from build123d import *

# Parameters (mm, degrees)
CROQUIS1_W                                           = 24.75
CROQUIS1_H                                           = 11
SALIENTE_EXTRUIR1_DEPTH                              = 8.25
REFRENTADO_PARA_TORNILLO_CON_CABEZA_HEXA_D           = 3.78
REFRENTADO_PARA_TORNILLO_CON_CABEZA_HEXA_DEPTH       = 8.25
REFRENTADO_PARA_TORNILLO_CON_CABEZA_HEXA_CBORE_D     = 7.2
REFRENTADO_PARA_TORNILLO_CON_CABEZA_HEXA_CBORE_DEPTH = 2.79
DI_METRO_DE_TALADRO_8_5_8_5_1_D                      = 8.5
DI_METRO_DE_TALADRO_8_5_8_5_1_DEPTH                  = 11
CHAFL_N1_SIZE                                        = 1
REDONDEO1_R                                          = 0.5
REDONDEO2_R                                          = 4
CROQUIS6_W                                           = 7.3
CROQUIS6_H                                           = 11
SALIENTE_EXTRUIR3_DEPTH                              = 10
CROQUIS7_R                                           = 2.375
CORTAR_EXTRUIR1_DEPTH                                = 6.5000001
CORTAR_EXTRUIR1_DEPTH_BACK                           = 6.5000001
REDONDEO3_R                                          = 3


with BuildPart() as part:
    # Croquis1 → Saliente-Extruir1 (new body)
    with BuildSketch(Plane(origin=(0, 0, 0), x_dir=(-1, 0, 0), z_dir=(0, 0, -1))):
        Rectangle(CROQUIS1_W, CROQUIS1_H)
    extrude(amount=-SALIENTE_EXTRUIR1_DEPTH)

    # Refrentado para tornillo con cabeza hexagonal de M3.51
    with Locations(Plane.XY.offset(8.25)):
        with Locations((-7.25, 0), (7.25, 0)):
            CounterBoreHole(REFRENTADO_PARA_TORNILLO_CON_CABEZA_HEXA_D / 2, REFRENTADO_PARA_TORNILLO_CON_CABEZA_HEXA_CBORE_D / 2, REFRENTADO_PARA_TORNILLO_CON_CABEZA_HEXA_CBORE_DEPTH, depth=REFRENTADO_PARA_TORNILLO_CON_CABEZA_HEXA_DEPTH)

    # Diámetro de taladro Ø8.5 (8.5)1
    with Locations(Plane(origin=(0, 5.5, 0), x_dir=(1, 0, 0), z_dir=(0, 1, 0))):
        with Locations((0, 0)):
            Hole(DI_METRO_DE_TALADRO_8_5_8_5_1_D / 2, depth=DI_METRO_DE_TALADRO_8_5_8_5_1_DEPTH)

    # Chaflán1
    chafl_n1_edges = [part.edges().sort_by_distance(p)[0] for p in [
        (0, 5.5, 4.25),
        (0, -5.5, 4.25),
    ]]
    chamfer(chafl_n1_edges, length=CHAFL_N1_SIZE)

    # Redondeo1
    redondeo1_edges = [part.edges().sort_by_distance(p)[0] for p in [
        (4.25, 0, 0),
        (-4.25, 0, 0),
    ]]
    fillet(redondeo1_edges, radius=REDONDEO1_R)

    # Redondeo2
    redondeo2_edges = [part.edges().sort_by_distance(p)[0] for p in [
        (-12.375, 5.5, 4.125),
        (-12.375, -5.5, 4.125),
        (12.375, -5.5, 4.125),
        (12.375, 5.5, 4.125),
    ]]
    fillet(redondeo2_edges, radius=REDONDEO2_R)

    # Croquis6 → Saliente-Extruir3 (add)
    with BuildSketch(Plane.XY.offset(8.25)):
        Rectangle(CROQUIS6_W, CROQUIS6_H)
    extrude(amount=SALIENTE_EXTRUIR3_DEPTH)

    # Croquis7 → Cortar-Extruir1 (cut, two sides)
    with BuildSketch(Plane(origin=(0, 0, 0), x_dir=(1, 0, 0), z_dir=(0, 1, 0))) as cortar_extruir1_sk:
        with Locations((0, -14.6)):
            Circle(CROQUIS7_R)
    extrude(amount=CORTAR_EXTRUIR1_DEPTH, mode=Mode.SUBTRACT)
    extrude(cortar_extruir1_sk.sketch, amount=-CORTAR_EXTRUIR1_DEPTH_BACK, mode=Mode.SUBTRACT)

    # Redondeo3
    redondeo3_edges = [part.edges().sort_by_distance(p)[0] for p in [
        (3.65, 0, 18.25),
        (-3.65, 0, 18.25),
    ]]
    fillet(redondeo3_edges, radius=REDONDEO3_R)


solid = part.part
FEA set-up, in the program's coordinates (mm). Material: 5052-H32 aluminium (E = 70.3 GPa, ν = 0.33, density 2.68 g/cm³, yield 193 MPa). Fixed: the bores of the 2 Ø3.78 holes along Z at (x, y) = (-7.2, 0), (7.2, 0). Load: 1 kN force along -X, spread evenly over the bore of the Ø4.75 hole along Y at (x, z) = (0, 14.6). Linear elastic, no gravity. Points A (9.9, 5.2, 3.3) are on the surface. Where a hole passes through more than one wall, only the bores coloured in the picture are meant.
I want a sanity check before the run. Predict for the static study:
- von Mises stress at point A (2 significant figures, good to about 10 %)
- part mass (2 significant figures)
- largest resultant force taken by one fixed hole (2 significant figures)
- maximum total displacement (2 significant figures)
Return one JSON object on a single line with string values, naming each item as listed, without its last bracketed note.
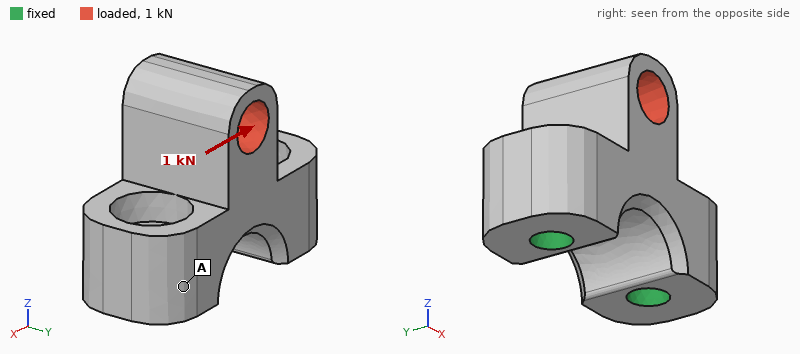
{"von Mises stress at point A": "9.5 MPa", "part mass": "5.4 g", "largest resultant force taken by one fixed hole": "1.1 kN", "maximum total displacement": "38 µm"}
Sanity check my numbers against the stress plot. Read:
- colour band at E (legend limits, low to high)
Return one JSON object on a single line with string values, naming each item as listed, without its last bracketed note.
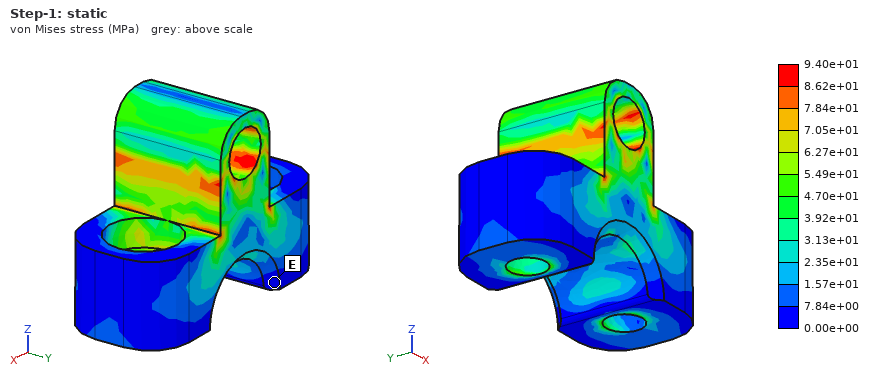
{"colour band at E": "0.00e+00 to 7.84e+00 MPa"}
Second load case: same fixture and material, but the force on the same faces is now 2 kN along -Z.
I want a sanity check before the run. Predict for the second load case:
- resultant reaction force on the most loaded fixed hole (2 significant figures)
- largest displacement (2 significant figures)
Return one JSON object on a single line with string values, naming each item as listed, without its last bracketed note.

{"resultant reaction force on the most loaded fixed hole": "1.1 kN", "largest displacement": "13 µm"}
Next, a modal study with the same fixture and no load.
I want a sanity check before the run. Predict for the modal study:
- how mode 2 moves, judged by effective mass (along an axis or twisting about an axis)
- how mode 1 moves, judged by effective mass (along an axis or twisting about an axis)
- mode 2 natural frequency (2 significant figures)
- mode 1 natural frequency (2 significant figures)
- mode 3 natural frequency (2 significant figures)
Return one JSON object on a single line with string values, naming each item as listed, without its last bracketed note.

{"how mode 2 moves, judged by effective mass": "along X", "how mode 1 moves, judged by effective mass": "along Y", "mode 2 natural frequency": "31 kHz", "mode 1 natural frequency": "24 kHz", "mode 3 natural frequency": "59 kHz"}
